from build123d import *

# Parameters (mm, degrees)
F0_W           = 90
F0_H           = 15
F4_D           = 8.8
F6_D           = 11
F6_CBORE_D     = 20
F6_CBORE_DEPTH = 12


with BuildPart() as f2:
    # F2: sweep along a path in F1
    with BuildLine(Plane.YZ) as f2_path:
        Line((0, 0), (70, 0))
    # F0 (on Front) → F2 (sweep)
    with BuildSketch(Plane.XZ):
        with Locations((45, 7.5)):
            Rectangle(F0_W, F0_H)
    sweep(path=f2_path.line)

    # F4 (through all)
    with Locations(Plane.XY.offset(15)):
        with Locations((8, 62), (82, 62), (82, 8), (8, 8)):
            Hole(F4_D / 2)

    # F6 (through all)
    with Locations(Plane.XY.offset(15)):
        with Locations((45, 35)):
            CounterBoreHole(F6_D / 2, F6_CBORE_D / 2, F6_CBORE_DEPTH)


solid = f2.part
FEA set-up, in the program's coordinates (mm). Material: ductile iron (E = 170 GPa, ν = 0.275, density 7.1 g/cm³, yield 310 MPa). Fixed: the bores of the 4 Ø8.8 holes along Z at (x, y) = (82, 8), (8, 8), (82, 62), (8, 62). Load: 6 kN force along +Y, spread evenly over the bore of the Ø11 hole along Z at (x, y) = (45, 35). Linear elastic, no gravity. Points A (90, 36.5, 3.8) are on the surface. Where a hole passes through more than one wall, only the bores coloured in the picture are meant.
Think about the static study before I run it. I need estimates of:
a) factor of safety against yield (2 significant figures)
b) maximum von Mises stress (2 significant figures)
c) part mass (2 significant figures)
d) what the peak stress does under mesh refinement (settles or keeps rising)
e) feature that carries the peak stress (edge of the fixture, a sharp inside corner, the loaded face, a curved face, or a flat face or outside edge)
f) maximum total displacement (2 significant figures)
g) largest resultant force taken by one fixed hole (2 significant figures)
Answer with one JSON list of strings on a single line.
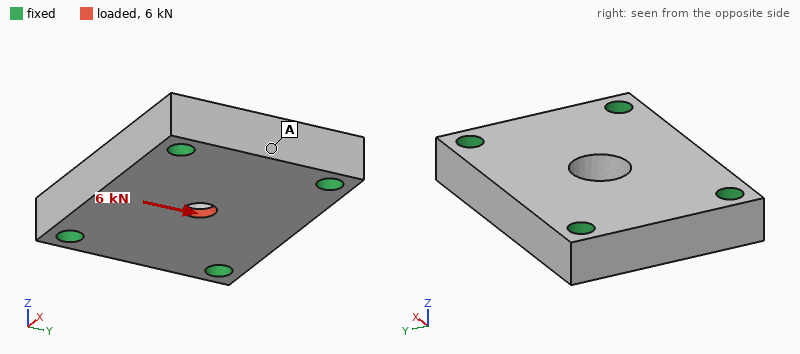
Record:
["2.9", "110 MPa", "620 g", "settles", "the loaded face", "5.2 µm", "1.8 kN"]
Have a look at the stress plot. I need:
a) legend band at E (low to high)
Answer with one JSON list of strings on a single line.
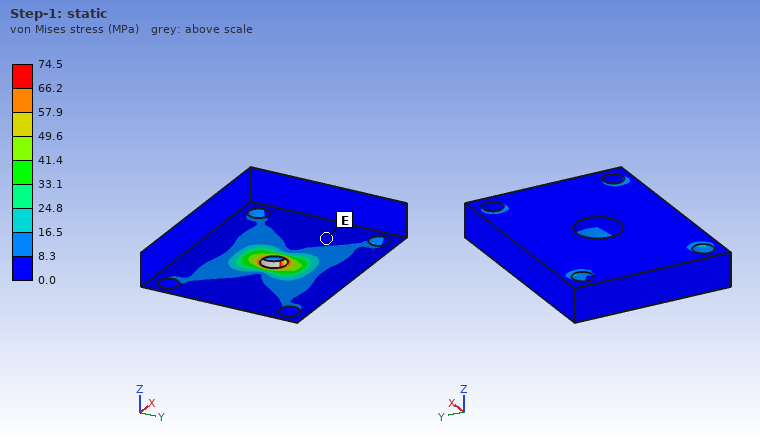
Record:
["0.0 to 8.3 MPa"]
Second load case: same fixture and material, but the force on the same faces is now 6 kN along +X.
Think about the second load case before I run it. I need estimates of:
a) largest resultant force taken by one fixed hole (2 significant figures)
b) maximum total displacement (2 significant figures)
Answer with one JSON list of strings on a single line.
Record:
["1.6 kN", "4.5 µm"]
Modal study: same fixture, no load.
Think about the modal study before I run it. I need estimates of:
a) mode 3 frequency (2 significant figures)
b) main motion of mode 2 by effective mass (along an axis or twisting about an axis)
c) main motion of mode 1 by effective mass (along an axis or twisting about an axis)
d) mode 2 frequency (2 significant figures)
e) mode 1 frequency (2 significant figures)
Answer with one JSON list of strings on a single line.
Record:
["19 kHz", "twisting about X", "along Z", "14 kHz", "10 kHz"]
